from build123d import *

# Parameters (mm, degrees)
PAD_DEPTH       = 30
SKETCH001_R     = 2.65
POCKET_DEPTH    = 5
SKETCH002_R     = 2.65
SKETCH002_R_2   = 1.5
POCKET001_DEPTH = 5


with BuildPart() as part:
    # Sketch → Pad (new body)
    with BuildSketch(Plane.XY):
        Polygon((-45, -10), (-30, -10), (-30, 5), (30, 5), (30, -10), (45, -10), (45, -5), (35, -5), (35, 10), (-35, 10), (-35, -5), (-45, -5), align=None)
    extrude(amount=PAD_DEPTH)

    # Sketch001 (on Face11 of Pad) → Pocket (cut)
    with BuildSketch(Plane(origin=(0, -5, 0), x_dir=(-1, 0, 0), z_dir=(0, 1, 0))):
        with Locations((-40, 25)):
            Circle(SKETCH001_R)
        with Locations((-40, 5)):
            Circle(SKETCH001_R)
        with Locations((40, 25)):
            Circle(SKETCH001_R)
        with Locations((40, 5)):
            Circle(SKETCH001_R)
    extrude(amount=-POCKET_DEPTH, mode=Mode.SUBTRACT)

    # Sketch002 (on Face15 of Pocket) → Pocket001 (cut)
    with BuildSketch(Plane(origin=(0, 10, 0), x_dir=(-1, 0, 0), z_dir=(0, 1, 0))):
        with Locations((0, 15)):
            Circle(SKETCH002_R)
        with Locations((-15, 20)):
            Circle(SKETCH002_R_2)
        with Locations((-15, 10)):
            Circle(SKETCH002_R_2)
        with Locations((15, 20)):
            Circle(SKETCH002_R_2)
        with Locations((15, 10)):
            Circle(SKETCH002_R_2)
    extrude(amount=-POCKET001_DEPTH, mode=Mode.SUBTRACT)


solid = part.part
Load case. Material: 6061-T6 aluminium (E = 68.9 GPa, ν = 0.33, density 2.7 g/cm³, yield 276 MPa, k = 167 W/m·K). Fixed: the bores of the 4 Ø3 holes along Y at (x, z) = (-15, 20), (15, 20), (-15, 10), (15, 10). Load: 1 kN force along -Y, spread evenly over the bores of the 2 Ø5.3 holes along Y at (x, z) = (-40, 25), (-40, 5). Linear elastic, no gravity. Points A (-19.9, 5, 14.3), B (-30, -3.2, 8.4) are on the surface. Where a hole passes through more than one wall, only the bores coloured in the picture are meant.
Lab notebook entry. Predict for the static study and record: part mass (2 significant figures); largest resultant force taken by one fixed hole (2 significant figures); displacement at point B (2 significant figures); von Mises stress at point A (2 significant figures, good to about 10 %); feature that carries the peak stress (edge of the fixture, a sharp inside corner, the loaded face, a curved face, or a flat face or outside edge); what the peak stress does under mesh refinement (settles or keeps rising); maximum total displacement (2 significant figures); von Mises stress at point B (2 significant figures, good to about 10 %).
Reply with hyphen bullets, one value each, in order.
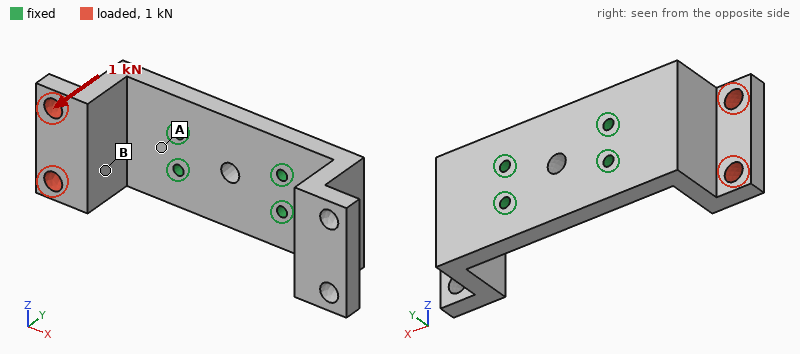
- 47 g
- 590 N
- 0.19 mm
- 150 MPa
- edge of the fixture
- keeps rising
- 0.46 mm
- 48 MPa
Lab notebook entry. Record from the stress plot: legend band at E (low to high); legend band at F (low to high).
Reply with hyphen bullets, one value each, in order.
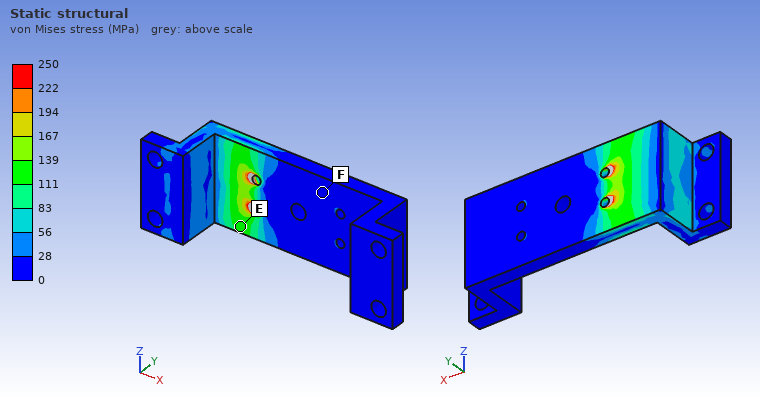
- 111 to 139 MPa
- 0 to 28 MPa
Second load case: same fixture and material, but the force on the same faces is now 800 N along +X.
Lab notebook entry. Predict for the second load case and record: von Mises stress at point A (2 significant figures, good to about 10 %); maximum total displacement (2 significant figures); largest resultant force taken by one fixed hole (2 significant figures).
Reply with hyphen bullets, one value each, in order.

- 93 MPa
- 0.32 mm
- 370 N
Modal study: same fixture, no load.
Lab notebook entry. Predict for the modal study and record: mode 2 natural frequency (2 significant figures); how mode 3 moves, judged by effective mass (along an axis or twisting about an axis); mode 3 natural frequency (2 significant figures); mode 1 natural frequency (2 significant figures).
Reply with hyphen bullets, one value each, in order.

- 2900 Hz
- twisting about Y
- 5300 Hz
- 2900 Hz
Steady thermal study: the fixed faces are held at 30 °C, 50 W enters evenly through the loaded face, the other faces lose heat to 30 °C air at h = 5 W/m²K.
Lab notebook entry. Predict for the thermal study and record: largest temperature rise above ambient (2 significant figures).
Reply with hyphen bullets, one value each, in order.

- 82 K
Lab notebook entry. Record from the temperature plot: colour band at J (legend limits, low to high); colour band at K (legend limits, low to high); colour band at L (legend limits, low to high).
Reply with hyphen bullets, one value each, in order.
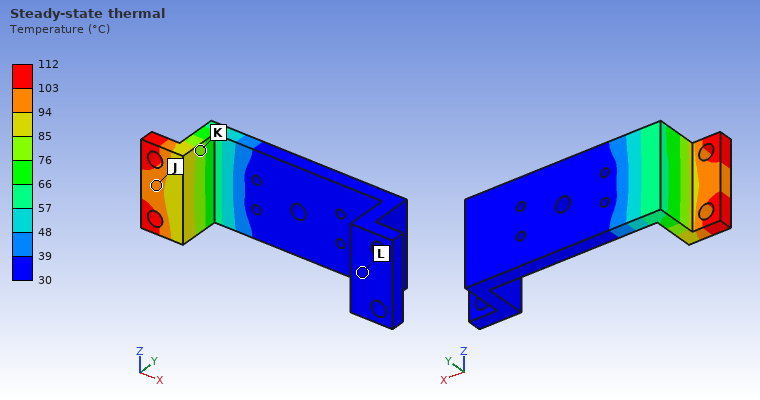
- 94 to 103 °C
- 76 to 85 °C
- 30 to 39 °C
